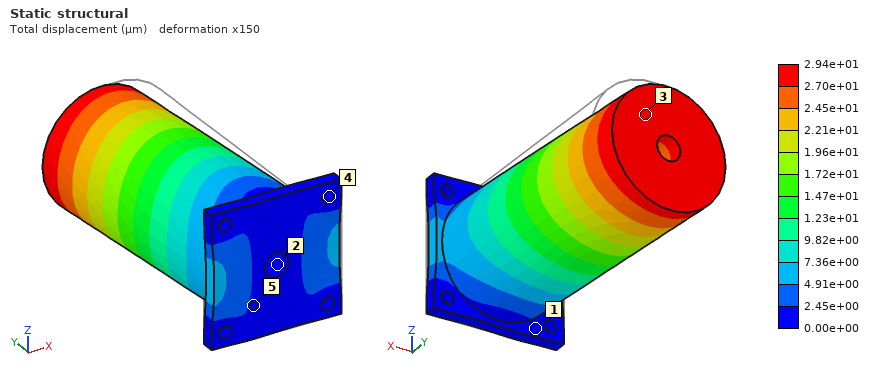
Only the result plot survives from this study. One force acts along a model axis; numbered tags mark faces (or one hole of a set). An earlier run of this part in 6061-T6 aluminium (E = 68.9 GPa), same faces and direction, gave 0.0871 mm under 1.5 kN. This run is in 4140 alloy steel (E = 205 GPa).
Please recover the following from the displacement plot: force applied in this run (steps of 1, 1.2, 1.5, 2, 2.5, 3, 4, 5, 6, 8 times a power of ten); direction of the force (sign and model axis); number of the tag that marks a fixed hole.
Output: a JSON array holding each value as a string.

["1.5 kN", "-X", "4"]
